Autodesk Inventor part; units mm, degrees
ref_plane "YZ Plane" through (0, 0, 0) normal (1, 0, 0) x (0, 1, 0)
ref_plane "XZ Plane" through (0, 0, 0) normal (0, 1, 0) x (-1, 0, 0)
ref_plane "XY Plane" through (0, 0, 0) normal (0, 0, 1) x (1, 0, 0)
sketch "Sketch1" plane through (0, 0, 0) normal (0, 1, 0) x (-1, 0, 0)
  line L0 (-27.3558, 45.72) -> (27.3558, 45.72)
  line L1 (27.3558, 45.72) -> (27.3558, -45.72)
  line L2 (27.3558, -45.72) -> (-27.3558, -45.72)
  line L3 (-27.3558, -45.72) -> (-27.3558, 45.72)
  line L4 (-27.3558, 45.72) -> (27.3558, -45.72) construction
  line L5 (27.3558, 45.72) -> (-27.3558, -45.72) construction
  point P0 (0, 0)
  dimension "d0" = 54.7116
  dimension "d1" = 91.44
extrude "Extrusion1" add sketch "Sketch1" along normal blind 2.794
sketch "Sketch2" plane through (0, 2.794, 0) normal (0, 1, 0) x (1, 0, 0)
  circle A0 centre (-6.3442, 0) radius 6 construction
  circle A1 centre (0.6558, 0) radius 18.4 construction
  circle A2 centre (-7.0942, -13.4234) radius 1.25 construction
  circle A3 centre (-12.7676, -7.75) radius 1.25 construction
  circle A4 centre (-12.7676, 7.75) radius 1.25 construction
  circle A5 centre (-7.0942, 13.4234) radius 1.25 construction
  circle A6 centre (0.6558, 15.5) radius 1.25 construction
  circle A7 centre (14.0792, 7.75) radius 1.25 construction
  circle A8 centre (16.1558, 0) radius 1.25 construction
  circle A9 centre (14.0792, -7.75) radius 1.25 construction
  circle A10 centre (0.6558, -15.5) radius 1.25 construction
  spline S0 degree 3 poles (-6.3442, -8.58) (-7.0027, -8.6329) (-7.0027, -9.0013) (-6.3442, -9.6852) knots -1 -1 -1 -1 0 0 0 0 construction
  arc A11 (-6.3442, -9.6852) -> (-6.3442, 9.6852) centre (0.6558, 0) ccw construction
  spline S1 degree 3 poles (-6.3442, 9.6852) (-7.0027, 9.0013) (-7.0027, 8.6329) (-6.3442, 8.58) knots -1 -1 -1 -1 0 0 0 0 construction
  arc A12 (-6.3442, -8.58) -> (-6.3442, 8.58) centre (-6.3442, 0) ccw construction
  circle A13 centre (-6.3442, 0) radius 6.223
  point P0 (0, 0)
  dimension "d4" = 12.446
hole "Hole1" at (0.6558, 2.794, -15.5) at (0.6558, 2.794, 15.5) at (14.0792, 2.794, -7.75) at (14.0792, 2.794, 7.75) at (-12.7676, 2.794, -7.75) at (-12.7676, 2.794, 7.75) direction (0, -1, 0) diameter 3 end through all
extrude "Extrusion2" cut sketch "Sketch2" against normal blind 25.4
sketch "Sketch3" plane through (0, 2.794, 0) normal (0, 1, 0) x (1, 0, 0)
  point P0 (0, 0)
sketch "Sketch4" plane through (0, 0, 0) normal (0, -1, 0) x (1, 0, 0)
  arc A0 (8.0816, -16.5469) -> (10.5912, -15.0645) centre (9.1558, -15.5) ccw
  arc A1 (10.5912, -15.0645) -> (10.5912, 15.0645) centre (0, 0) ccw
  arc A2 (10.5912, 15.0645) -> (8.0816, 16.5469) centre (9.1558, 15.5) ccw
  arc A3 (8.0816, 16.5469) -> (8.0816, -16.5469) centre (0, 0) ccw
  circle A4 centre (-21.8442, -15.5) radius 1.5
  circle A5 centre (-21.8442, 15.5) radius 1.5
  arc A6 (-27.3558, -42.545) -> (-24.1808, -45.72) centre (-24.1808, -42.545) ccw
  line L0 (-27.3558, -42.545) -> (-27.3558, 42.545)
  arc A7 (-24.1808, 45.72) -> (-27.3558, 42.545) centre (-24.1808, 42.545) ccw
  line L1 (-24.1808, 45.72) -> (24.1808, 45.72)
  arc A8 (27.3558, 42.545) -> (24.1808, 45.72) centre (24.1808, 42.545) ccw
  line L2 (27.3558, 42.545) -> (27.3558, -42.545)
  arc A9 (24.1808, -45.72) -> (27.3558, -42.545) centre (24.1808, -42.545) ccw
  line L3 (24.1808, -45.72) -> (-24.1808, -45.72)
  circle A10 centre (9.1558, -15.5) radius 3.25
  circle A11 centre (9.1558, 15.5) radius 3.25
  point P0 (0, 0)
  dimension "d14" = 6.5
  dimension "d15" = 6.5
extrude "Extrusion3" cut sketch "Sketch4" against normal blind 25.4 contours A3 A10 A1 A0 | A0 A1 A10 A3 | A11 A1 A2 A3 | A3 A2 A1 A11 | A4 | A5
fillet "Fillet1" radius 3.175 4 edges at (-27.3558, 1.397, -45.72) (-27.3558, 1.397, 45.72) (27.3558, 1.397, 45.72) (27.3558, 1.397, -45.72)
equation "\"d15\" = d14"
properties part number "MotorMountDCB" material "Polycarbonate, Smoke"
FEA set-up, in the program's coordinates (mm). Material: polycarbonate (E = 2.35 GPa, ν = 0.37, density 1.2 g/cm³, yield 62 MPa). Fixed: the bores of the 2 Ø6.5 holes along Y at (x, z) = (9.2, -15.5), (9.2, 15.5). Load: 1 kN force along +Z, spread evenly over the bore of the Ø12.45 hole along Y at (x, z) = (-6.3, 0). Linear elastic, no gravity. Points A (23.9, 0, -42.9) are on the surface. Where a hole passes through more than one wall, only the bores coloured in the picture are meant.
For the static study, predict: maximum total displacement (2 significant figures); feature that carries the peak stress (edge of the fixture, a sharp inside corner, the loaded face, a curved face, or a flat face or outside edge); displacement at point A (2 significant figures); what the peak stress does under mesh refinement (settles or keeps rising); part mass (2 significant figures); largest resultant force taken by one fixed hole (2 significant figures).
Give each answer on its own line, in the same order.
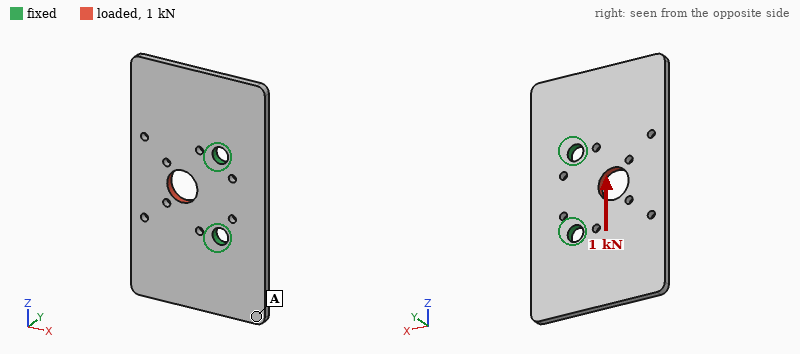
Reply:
0.35 mm
edge of the fixture
0.19 mm
keeps rising
16 g
640 N
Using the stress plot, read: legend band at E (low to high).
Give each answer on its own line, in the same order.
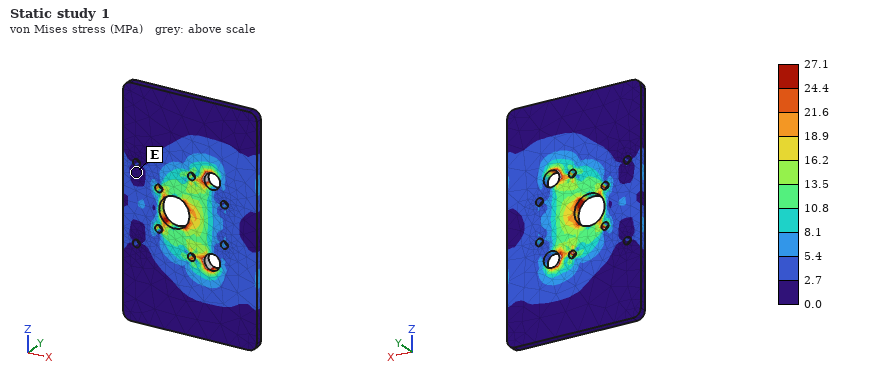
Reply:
0.0 to 2.7 MPa
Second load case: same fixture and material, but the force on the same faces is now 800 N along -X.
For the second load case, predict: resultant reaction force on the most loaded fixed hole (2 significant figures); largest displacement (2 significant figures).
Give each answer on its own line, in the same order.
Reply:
420 N
0.11 mm
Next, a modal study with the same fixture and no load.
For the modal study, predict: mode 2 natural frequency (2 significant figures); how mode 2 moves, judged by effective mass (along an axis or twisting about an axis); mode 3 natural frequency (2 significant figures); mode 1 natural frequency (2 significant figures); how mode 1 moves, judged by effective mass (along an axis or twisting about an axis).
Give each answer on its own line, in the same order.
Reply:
460 Hz
twisting about X
680 Hz
420 Hz
along Y
